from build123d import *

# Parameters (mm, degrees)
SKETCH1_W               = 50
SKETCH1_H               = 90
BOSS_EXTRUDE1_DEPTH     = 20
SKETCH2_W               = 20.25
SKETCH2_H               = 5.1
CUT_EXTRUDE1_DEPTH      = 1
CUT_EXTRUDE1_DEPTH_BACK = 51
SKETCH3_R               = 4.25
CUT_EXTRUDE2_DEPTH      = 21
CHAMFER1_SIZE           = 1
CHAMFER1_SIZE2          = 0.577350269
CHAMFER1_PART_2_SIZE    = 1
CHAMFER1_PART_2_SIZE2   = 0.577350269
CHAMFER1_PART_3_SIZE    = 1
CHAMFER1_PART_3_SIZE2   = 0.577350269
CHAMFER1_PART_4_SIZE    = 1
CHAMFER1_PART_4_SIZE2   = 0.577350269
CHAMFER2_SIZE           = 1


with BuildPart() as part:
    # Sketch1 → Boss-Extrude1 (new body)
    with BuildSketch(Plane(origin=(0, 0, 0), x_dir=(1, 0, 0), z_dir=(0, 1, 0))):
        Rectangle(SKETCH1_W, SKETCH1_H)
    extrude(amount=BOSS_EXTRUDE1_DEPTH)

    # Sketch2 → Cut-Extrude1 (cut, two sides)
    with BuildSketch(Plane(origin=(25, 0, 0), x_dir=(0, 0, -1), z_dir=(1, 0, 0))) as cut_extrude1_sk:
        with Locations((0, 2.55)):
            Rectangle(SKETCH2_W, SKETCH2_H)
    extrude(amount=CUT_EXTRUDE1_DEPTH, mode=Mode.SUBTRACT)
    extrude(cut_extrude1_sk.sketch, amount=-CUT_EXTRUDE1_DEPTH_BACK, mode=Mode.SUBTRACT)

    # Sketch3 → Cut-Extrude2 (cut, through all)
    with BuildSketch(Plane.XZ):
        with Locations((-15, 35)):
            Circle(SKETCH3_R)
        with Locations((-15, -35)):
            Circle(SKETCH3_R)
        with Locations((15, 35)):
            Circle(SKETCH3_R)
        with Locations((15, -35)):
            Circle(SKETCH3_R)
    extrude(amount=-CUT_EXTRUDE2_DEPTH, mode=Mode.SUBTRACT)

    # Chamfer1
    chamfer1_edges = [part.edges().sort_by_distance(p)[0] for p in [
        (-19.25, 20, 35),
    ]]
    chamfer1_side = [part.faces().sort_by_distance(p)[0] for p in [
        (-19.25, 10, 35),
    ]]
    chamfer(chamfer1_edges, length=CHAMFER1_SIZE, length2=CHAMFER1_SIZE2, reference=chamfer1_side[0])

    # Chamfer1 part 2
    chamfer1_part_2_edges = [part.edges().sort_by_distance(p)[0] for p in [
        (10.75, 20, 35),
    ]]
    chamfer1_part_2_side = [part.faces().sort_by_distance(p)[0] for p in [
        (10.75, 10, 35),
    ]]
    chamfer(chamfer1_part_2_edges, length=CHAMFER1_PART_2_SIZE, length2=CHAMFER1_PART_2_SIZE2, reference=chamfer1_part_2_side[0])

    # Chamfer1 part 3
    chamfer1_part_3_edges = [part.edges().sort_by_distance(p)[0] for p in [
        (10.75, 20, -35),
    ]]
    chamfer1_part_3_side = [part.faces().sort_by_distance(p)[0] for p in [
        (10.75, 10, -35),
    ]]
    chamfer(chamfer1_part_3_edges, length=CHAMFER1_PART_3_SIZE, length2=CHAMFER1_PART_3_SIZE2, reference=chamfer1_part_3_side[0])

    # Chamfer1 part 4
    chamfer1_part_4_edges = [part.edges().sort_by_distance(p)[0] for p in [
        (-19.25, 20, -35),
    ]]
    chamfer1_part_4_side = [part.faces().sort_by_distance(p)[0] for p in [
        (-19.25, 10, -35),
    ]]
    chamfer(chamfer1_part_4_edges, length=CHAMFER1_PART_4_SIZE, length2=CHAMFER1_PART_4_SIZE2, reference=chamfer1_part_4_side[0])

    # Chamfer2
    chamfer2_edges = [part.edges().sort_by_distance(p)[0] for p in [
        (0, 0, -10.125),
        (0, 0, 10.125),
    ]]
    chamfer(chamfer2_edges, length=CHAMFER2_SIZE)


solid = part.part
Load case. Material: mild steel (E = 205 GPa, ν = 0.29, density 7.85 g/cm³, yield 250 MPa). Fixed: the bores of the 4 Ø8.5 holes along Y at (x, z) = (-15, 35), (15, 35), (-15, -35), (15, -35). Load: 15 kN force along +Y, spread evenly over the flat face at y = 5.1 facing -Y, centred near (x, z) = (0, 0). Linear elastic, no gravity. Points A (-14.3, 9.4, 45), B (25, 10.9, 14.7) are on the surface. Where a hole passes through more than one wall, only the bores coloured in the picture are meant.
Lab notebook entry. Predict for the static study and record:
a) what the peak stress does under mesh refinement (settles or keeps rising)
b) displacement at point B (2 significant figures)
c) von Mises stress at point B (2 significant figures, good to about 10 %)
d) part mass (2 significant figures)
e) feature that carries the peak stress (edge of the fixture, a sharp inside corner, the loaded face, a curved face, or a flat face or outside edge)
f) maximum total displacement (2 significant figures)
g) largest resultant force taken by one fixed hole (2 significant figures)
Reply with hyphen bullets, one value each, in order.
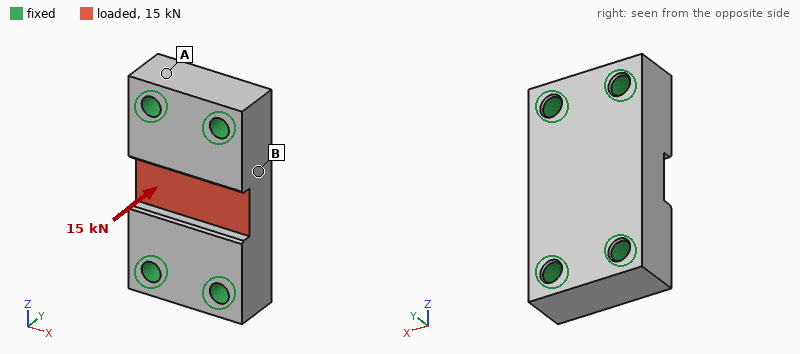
- keeps rising
- 4.9 µm
- 27 MPa
- 630 g
- edge of the fixture
- 8.9 µm
- 4.0 kN
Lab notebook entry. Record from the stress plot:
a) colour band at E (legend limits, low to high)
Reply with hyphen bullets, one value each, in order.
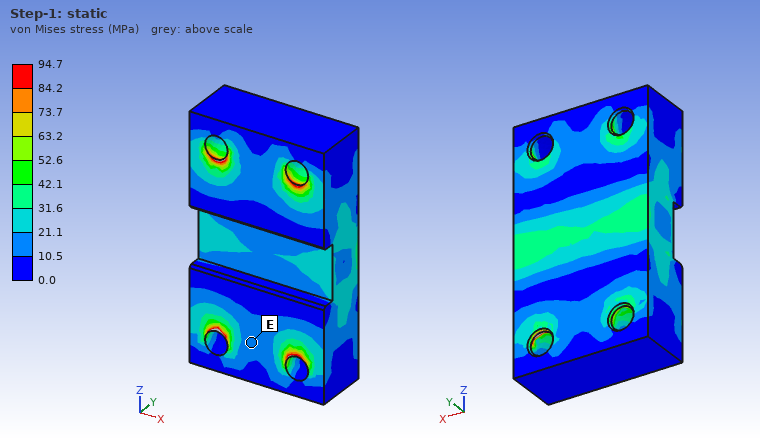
- 10.5 to 21.1 MPa
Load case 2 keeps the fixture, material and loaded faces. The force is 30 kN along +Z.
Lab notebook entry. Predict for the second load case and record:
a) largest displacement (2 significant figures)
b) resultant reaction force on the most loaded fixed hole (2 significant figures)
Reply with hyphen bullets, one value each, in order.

- 4.8 µm
- 7.7 kN
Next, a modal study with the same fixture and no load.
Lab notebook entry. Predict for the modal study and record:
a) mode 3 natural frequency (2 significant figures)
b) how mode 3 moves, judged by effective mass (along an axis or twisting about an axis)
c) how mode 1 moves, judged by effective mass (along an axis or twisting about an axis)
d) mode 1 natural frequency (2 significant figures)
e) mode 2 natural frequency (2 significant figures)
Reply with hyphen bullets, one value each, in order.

- 22 kHz
- along X
- along Y
- 15 kHz
- 20 kHz
